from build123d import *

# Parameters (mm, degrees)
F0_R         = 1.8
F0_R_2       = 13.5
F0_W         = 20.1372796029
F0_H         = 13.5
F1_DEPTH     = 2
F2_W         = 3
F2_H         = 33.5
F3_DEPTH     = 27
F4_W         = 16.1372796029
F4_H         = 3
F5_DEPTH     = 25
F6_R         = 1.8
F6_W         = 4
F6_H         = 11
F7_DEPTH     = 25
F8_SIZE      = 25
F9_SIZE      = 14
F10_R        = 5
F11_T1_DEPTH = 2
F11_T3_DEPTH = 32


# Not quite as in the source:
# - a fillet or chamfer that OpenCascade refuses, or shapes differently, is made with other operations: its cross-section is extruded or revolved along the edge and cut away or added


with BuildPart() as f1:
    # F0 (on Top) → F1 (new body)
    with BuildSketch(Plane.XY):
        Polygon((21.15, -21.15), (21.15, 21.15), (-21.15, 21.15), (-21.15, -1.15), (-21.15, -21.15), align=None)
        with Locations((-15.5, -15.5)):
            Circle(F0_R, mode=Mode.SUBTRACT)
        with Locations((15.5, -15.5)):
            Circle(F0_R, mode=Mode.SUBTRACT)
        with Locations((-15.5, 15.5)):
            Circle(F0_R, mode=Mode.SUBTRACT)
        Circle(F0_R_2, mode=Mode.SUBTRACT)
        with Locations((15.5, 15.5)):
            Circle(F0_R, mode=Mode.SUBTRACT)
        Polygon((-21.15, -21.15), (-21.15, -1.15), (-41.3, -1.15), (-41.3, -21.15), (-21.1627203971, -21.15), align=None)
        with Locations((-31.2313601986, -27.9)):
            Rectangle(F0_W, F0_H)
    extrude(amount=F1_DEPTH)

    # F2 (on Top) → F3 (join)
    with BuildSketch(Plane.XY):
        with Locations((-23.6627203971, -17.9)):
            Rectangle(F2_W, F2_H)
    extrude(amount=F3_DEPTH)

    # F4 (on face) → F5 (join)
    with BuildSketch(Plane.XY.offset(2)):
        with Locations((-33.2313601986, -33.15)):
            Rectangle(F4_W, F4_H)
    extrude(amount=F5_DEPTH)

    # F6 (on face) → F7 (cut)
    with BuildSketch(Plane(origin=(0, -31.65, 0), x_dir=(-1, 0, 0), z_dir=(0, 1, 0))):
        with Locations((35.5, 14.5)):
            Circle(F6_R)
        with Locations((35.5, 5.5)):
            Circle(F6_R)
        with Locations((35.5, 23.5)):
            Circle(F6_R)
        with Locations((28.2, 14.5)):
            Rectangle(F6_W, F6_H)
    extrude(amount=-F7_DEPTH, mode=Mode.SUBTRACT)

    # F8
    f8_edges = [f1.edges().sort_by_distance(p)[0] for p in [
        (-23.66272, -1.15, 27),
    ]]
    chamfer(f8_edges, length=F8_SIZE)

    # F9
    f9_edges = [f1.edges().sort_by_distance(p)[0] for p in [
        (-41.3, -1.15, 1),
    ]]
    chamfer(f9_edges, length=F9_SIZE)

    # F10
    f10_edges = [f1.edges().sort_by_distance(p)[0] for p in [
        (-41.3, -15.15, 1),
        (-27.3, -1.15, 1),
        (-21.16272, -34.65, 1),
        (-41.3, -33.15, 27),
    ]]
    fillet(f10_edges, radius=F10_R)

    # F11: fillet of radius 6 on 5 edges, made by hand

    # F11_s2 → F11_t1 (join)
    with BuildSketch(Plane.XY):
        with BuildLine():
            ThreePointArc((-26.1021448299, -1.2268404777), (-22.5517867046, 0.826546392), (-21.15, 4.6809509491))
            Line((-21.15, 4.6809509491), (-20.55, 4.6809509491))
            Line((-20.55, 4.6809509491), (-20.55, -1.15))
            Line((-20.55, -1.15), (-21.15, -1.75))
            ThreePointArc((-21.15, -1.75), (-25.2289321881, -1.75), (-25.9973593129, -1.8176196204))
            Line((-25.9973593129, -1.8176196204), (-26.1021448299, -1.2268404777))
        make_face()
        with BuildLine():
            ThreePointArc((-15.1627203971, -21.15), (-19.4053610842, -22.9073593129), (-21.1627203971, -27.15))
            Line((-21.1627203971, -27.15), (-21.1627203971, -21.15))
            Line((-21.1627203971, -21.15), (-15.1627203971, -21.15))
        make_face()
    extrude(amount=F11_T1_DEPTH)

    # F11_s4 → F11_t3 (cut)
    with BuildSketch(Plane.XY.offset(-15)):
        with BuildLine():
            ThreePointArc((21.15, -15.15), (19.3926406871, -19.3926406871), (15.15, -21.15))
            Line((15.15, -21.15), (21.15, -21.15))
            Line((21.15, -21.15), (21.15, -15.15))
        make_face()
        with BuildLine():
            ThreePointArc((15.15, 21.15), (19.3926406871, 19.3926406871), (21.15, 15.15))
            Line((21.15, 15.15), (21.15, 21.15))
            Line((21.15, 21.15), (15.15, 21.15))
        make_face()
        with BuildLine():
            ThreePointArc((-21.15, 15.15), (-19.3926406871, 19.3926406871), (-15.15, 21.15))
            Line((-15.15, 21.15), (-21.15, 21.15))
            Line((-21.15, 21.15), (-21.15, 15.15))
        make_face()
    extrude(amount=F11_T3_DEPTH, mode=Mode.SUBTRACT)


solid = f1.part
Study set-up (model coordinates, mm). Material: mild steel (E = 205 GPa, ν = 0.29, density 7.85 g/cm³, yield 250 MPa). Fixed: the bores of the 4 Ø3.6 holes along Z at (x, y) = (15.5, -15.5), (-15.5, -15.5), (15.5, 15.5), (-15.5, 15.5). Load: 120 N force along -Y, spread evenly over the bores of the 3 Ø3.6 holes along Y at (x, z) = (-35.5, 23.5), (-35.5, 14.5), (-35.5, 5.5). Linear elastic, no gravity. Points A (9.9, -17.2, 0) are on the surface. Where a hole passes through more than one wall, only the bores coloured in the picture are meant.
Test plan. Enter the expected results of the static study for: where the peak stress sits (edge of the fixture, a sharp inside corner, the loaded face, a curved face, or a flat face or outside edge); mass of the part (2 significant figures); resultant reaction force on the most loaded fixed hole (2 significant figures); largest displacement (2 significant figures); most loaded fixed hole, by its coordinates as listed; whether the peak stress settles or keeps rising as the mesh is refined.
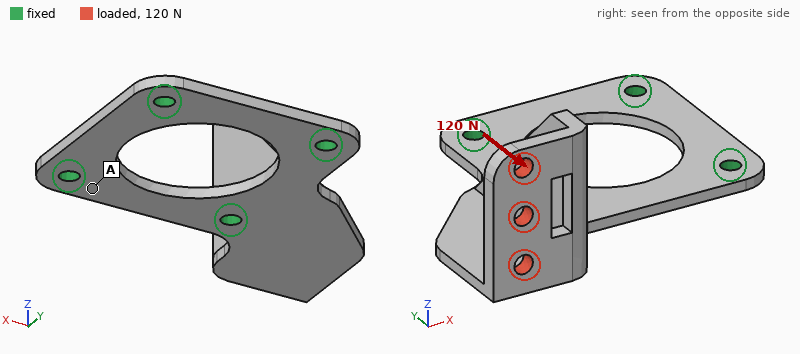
edge of the fixture
47 g
120 N
52 µm
(-15.5, 15.5)
keeps rising
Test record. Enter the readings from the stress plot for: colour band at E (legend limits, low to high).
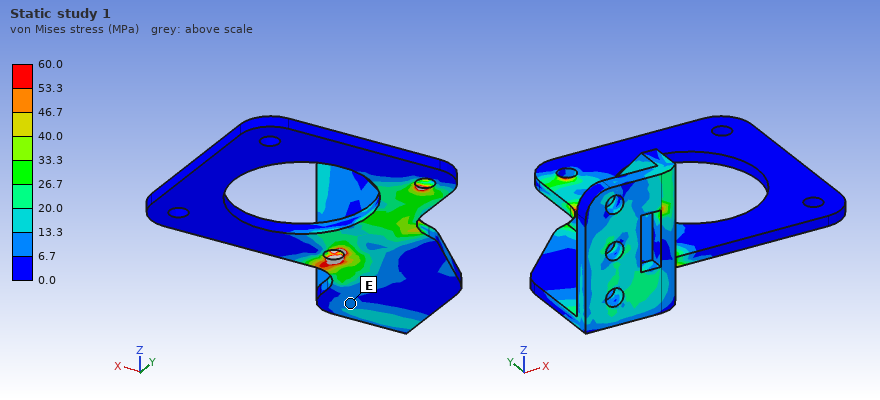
6.7 to 13.3 MPa
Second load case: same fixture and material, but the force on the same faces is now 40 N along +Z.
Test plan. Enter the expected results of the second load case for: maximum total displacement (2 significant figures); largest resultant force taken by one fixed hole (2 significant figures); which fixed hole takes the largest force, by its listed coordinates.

73 µm
57 N
(-15.5, -15.5)
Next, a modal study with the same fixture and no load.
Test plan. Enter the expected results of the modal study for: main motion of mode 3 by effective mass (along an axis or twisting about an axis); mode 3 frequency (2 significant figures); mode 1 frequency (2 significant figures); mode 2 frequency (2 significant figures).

along Z
6100 Hz
1100 Hz
2200 Hz
